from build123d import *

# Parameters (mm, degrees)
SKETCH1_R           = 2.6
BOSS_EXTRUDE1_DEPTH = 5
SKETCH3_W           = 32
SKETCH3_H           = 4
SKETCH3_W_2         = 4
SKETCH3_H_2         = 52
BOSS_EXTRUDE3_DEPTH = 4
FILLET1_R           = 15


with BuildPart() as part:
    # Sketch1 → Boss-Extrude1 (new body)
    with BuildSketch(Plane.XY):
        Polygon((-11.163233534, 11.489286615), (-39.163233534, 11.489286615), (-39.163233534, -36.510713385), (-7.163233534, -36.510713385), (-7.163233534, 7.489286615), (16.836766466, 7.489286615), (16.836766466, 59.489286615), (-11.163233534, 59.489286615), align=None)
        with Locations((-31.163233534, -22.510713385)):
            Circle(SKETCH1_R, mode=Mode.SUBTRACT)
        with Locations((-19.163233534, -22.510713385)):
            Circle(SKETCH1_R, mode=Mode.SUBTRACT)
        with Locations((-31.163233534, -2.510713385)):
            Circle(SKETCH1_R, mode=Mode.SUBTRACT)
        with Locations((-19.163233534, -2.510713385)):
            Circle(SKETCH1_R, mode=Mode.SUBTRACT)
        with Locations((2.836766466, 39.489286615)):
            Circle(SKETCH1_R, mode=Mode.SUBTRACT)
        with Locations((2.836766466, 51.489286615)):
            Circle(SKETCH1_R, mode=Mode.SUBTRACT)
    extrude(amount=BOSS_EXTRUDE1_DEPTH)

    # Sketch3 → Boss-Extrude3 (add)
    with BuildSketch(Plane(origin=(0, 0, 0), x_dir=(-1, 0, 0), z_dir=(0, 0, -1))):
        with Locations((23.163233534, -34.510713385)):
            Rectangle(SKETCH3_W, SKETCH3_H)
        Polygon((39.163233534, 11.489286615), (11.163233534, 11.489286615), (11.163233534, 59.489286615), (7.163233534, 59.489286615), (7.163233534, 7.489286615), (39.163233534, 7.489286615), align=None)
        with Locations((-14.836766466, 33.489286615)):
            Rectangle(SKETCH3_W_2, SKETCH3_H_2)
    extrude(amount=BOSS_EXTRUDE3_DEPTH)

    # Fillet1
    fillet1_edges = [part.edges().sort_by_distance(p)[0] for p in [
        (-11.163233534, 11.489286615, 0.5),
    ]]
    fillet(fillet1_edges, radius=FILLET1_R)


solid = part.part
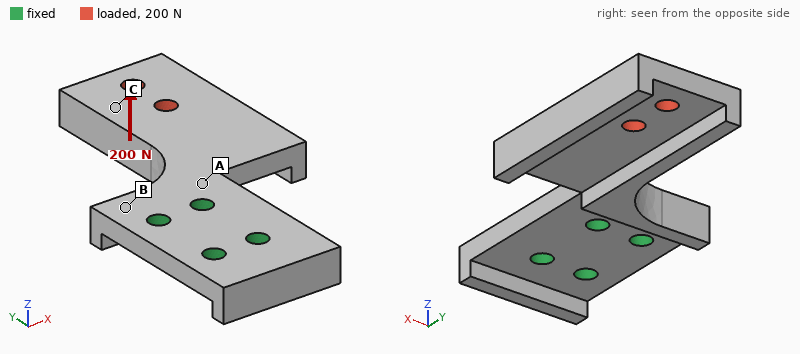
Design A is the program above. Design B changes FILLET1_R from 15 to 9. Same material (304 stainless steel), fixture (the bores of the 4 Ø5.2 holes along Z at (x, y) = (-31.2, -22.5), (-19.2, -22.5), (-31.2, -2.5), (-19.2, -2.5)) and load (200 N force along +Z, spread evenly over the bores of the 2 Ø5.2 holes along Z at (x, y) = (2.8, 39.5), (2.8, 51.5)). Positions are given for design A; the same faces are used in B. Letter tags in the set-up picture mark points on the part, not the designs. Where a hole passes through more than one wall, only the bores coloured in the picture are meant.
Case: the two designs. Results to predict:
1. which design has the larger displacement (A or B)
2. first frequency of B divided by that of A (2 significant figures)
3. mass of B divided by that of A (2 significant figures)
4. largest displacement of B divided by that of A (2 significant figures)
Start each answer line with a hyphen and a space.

- B
- 0.93
- 0.98
- 1.2
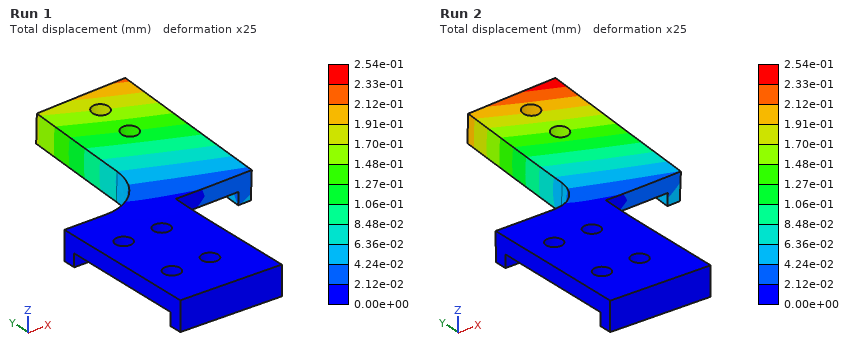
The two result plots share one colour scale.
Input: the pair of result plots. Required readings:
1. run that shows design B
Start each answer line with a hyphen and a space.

- Run 2
